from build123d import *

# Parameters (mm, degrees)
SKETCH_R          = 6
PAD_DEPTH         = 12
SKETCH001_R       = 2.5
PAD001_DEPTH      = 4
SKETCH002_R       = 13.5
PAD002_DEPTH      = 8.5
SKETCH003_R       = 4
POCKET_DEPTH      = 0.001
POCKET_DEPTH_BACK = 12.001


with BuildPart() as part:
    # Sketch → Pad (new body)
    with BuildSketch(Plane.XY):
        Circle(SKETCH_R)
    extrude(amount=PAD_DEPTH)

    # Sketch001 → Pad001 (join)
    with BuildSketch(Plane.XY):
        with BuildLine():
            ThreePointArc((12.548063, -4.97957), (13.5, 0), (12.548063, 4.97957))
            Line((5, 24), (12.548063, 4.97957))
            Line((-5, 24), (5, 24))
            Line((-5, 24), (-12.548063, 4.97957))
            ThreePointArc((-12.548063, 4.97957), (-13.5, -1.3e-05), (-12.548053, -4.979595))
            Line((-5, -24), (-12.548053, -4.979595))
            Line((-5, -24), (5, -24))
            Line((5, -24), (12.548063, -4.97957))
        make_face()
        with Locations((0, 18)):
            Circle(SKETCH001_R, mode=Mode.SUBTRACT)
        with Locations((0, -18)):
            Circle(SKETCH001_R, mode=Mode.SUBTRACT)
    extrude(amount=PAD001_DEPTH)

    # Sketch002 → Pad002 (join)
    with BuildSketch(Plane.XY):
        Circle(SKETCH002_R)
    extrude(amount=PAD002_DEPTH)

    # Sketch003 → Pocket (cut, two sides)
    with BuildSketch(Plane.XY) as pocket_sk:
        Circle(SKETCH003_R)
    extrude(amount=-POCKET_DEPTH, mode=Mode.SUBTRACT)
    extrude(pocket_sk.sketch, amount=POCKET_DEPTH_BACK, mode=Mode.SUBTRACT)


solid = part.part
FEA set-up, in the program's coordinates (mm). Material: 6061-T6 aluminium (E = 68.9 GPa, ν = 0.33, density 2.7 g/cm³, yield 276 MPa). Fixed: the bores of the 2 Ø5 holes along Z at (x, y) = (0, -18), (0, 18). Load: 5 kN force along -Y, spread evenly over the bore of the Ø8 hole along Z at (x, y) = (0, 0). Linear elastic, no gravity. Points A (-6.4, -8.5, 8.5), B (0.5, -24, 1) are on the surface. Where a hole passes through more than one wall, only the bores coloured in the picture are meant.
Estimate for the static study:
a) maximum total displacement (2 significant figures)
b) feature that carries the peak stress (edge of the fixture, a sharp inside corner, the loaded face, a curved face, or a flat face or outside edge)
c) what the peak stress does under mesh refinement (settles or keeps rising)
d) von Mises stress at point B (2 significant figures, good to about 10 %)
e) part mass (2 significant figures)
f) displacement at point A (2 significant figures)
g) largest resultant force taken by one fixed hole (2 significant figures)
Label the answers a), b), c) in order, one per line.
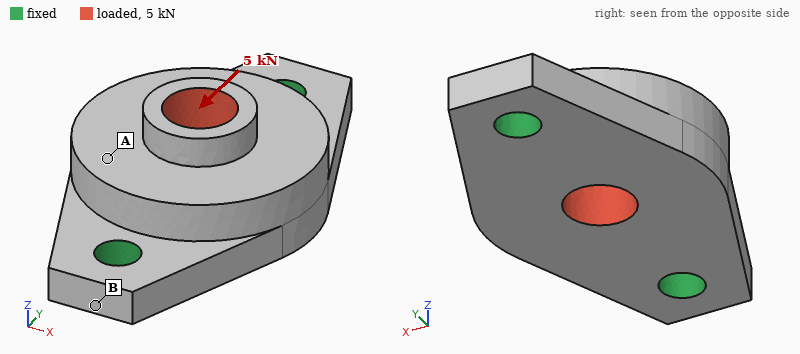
a) 16 µm
b) edge of the fixture
c) keeps rising
d) 24 MPa
e) 16 g
f) 7.7 µm
g) 2.6 kN
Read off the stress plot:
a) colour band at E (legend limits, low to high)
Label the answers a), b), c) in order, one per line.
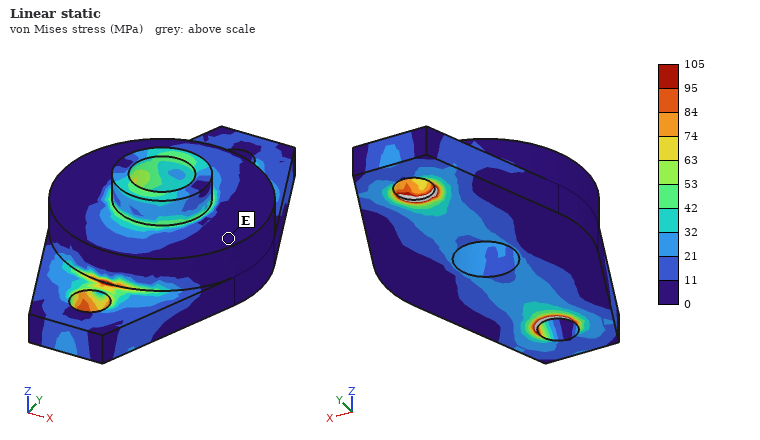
a) 0 to 11 MPa
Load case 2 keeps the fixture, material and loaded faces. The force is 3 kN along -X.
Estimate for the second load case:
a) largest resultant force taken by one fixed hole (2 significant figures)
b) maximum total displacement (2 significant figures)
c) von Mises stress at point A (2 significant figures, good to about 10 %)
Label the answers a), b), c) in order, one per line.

a) 1.5 kN
b) 54 µm
c) 21 MPa
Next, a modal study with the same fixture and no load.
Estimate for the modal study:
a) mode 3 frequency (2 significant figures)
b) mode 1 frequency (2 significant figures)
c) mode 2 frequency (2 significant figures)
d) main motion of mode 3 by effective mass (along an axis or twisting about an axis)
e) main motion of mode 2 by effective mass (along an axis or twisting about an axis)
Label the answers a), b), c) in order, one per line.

a) 28 kHz
b) 11 kHz
c) 16 kHz
d) along X
e) along Z
